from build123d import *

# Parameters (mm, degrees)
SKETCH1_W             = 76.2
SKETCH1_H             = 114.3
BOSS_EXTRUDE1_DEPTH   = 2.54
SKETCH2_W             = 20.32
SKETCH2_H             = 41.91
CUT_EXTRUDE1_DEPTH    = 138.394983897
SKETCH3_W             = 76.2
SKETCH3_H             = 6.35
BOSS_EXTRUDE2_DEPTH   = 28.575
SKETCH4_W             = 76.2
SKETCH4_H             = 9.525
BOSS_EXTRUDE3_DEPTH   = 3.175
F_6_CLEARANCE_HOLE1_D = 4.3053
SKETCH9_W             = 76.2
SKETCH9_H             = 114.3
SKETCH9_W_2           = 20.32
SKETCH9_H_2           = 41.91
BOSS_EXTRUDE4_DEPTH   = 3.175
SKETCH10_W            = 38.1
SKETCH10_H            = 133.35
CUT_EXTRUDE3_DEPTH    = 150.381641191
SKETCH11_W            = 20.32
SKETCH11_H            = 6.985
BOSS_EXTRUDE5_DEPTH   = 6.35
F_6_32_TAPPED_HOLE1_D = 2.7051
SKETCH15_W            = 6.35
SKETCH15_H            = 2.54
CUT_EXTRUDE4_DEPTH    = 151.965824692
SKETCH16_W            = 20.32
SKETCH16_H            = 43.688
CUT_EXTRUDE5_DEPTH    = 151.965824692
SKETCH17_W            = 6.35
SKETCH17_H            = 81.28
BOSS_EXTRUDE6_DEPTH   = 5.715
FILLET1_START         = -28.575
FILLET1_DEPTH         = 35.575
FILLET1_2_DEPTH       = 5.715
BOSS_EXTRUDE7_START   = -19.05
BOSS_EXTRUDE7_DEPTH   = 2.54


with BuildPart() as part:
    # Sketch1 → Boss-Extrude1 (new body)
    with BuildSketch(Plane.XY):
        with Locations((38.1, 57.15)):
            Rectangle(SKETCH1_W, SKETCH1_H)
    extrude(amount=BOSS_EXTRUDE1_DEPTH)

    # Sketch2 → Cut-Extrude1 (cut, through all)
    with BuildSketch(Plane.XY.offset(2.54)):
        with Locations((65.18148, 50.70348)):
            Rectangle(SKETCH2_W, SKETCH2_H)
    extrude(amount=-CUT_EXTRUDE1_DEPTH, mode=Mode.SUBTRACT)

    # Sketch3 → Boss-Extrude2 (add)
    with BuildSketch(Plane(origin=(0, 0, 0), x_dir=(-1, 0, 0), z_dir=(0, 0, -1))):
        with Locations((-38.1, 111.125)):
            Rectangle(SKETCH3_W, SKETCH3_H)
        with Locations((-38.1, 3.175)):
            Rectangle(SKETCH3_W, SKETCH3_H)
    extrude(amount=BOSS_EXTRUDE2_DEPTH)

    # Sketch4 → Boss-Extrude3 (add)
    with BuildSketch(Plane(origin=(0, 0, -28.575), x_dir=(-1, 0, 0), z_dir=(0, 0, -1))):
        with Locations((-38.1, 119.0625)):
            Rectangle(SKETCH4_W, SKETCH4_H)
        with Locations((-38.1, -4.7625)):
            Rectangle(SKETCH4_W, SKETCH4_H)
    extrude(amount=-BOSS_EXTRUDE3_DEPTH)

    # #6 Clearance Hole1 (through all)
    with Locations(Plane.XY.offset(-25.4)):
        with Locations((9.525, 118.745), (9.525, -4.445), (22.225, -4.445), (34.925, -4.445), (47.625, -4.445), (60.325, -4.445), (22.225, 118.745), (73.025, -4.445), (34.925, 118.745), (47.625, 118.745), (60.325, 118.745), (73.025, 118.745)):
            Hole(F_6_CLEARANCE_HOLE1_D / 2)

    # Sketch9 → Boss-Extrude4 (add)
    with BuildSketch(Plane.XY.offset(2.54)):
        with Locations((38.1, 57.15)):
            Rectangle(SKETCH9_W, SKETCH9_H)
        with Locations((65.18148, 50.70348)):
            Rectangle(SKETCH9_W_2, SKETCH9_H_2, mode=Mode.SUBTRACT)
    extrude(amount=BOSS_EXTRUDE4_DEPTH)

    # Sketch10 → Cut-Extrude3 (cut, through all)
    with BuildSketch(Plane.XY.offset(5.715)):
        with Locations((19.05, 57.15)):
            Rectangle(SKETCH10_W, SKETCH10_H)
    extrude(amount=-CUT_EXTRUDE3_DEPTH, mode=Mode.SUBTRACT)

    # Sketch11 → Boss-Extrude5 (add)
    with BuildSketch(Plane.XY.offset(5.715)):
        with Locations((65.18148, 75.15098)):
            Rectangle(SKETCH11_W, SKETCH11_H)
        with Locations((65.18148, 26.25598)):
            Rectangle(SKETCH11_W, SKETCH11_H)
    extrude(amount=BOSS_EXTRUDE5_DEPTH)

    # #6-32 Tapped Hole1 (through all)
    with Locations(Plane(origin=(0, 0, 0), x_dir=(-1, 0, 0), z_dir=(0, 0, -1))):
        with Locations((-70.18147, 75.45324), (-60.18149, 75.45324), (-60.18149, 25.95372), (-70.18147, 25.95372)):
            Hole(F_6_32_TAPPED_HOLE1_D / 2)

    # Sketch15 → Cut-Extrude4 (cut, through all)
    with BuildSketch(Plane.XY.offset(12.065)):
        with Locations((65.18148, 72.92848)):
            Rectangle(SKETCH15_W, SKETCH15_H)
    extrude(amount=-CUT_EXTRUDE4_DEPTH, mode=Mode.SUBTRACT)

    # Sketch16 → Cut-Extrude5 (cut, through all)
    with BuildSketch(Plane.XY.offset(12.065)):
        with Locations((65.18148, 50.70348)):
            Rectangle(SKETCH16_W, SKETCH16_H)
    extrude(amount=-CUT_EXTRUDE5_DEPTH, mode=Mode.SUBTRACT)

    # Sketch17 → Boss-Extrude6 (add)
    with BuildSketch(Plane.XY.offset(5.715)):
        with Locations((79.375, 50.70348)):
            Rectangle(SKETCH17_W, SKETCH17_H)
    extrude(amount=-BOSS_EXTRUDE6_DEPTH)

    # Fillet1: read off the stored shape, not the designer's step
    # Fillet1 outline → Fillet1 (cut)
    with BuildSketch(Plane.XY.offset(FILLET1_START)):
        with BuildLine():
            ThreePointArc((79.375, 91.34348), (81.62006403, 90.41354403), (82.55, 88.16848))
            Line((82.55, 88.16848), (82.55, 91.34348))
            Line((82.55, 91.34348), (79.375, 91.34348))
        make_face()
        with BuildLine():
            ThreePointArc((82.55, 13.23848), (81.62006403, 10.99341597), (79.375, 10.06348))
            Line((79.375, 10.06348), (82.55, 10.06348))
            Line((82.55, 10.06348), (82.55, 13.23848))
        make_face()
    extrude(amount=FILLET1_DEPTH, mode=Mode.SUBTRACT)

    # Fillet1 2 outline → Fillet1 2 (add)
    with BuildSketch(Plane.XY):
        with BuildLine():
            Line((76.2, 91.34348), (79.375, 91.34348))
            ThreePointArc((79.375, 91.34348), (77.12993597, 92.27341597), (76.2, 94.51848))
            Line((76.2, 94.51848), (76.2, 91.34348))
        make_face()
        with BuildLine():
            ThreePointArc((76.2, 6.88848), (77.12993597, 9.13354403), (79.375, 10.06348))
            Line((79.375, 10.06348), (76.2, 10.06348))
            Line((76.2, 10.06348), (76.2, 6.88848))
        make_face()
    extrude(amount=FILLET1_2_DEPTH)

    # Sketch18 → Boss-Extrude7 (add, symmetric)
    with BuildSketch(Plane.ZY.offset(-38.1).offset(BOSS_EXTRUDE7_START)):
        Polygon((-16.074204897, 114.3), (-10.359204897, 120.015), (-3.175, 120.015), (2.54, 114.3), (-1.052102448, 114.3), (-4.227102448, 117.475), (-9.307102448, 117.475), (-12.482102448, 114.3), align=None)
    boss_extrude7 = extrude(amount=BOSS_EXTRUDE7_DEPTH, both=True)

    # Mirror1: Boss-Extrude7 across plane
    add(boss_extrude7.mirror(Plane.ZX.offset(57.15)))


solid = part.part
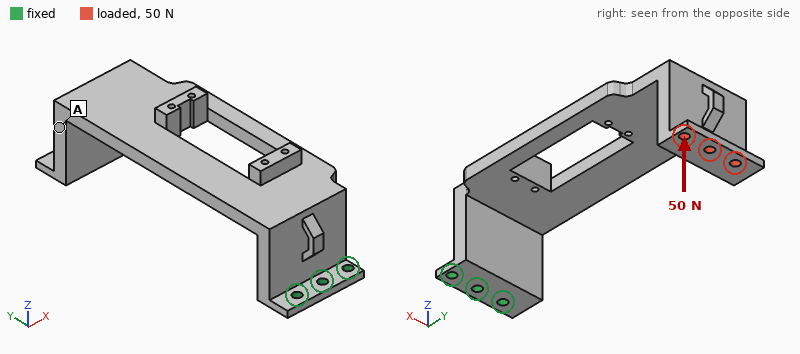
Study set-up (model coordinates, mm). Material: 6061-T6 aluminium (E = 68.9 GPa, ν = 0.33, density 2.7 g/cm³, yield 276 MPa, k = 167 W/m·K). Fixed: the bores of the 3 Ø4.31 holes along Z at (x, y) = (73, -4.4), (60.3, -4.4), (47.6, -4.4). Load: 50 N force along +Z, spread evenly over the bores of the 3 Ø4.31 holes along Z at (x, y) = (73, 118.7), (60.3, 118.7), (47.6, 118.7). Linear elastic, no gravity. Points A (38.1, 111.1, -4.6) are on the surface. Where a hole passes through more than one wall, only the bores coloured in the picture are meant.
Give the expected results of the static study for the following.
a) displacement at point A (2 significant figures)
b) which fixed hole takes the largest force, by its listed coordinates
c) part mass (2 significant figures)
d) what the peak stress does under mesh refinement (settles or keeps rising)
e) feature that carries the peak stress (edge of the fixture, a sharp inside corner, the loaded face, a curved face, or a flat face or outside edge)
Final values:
1.4 mm
(60.3, -4.4)
110 g
keeps rising
edge of the fixture
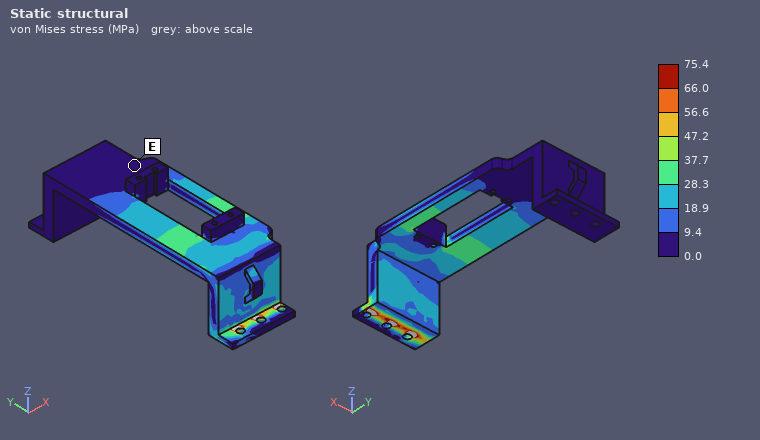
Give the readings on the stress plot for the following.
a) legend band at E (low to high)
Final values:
0.0 to 9.4 MPa
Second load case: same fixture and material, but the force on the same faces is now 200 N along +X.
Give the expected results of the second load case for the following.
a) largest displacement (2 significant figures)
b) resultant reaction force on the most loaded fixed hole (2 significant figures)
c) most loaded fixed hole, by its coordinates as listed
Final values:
1.5 mm
960 N
(47.6, -4.4)
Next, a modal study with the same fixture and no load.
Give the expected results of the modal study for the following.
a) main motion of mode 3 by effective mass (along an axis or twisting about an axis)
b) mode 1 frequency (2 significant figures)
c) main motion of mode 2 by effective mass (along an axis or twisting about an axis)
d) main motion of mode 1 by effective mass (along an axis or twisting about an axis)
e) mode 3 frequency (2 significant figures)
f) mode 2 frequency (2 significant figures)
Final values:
along Y
150 Hz
along X
along Z
680 Hz
360 Hz
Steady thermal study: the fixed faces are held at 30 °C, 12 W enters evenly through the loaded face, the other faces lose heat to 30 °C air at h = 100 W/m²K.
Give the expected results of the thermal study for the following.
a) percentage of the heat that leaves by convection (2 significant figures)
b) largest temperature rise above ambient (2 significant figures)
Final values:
92 %
23 K
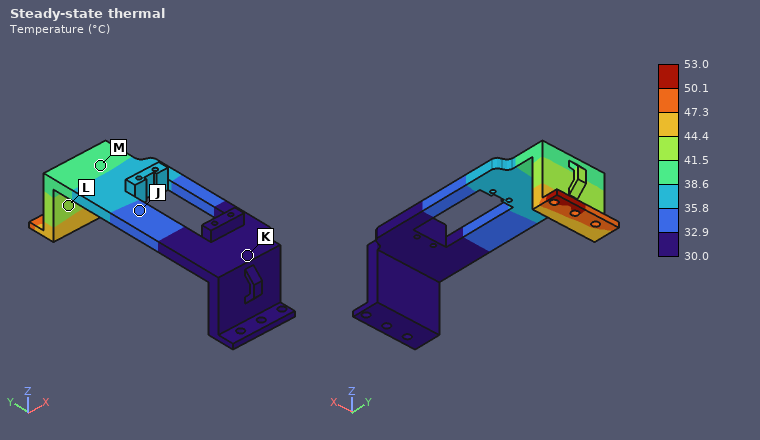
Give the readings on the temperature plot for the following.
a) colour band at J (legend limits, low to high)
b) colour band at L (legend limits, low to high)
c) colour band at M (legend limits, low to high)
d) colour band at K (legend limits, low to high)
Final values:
32.9 to 35.8 °C
41.5 to 44.4 °C
38.6 to 41.5 °C
30.0 to 32.9 °C
